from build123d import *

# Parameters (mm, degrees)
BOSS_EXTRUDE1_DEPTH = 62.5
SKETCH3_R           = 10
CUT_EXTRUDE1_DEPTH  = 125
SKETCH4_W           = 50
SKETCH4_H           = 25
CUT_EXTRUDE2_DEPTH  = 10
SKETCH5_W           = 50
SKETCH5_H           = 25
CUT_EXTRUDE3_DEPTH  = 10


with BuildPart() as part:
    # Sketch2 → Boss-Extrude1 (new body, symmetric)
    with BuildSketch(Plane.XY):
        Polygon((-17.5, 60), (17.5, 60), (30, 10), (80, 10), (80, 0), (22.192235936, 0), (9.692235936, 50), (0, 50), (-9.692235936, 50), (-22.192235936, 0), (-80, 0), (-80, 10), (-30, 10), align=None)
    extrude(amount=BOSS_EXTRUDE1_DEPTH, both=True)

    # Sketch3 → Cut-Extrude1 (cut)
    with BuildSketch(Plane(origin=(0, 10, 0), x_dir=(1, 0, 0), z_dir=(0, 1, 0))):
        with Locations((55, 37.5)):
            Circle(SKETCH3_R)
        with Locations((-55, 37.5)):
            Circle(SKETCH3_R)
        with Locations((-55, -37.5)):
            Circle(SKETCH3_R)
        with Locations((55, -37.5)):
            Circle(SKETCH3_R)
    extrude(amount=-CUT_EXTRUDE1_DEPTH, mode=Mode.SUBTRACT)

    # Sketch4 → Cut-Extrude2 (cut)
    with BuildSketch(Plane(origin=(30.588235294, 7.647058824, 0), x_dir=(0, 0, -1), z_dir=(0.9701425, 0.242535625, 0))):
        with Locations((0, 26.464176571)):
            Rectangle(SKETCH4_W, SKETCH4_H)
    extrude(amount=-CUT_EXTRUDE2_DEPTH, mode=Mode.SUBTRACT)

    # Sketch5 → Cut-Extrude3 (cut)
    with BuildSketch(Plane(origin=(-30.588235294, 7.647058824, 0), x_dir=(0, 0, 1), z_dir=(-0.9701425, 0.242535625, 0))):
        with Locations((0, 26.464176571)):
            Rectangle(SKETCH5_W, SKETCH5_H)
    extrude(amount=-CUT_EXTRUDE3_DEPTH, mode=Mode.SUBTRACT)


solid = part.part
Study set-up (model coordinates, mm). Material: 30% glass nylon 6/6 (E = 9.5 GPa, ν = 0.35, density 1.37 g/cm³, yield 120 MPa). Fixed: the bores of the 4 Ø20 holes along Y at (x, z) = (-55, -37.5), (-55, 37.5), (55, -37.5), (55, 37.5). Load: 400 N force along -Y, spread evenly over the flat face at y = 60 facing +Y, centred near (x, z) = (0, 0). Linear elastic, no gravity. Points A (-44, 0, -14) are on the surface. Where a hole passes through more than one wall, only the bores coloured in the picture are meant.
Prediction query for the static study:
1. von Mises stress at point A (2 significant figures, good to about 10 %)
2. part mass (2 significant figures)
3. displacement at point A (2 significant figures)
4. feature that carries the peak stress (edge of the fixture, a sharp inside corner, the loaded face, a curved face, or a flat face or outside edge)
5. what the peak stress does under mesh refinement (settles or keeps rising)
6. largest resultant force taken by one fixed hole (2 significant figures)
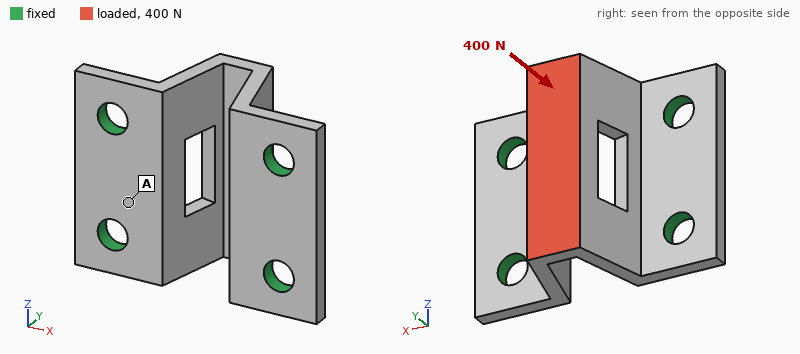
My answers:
0.38 MPa
360 g
1.8 µm
edge of the fixture
keeps rising
110 N
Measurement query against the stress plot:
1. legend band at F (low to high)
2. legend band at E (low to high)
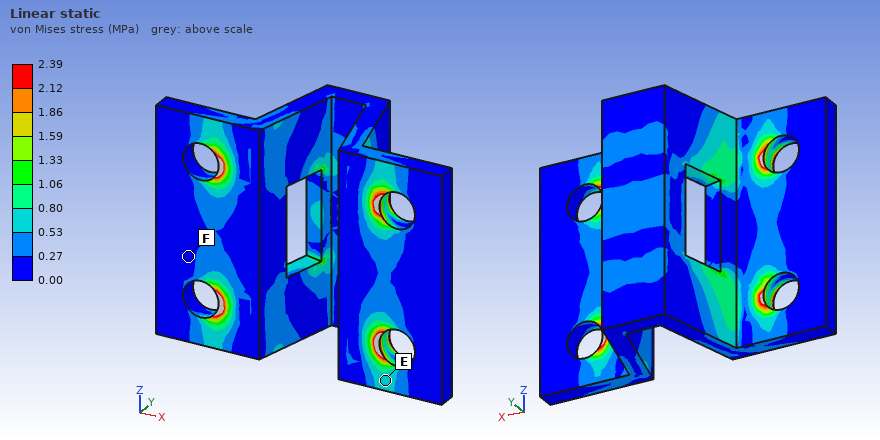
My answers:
0.00 to 0.27 MPa
0.53 to 0.80 MPa
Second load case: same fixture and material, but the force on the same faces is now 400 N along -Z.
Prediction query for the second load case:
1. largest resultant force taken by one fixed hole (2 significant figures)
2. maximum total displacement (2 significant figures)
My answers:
190 N
36 µm
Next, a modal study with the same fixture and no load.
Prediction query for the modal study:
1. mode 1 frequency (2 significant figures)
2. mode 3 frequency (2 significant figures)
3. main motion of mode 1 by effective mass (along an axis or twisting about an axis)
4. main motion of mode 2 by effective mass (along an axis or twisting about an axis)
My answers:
1800 Hz
2400 Hz
along Z
along X
